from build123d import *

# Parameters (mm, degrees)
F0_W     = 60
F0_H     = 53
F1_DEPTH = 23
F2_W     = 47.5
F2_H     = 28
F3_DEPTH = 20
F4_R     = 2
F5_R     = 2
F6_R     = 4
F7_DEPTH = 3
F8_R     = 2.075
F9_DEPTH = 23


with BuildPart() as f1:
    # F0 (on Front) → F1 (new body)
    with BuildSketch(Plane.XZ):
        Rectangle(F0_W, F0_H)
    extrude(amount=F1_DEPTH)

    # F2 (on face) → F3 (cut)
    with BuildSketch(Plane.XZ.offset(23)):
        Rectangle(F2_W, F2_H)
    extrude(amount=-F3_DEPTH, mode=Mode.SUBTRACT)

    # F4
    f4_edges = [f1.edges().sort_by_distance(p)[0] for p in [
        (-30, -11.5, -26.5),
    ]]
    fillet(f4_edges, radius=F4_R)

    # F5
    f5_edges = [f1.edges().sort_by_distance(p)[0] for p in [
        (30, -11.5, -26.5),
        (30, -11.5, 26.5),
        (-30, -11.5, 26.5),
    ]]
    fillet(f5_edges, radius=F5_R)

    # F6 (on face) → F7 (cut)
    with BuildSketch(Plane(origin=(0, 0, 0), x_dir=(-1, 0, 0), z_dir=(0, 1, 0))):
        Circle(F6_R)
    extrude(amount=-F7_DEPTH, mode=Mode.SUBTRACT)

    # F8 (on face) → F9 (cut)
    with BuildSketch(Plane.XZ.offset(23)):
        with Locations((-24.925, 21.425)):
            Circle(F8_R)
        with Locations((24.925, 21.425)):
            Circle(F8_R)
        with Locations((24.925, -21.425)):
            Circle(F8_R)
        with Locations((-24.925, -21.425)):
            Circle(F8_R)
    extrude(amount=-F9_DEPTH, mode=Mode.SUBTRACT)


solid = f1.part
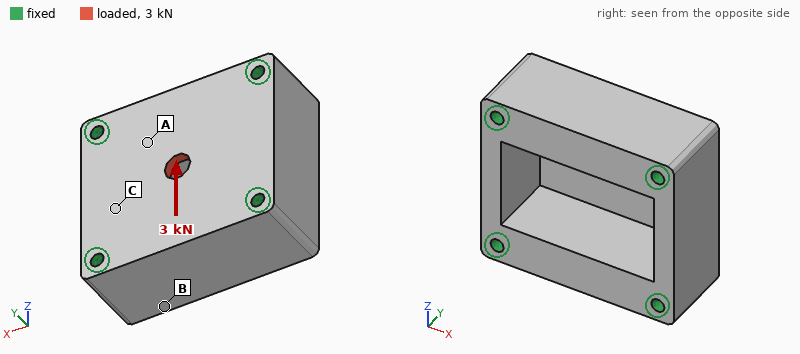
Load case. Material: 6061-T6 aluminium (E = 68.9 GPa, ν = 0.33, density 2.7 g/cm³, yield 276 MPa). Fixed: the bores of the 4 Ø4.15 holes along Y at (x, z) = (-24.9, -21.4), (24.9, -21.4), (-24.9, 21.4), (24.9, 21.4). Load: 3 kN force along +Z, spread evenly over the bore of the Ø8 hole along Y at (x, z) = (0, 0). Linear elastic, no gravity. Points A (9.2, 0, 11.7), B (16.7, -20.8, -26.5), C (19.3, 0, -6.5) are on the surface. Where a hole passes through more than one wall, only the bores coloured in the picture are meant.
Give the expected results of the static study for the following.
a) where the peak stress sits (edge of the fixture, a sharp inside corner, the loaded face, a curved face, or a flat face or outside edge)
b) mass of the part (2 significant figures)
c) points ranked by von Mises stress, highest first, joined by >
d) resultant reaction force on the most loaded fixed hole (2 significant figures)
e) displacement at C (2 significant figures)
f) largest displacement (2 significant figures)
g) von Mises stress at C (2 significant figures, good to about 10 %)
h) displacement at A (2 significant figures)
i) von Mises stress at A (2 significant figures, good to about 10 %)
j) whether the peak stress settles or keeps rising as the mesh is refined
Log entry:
a sharp inside corner
120 g
A > C > B
870 N
1.9 µm
10 µm
8.9 MPa
5.2 µm
17 MPa
keeps rising
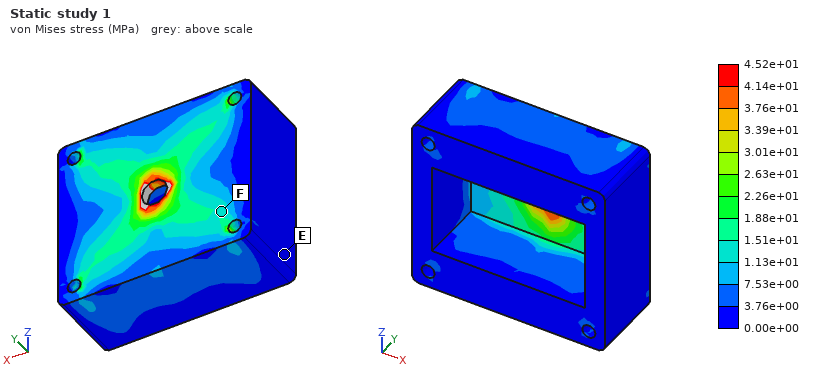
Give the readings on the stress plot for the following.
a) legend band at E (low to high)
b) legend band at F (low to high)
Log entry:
0.00e+00 to 3.76e+00 MPa
1.13e+01 to 1.51e+01 MPa
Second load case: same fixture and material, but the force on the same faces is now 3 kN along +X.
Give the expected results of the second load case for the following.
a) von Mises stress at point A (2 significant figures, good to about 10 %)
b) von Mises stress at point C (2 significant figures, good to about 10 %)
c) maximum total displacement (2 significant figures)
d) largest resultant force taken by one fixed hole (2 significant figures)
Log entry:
16 MPa
11 MPa
8.7 µm
840 N
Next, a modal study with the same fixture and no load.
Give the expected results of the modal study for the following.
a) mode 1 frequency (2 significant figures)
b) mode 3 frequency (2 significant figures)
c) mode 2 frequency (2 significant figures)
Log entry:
17 kHz
20 kHz
20 kHz
